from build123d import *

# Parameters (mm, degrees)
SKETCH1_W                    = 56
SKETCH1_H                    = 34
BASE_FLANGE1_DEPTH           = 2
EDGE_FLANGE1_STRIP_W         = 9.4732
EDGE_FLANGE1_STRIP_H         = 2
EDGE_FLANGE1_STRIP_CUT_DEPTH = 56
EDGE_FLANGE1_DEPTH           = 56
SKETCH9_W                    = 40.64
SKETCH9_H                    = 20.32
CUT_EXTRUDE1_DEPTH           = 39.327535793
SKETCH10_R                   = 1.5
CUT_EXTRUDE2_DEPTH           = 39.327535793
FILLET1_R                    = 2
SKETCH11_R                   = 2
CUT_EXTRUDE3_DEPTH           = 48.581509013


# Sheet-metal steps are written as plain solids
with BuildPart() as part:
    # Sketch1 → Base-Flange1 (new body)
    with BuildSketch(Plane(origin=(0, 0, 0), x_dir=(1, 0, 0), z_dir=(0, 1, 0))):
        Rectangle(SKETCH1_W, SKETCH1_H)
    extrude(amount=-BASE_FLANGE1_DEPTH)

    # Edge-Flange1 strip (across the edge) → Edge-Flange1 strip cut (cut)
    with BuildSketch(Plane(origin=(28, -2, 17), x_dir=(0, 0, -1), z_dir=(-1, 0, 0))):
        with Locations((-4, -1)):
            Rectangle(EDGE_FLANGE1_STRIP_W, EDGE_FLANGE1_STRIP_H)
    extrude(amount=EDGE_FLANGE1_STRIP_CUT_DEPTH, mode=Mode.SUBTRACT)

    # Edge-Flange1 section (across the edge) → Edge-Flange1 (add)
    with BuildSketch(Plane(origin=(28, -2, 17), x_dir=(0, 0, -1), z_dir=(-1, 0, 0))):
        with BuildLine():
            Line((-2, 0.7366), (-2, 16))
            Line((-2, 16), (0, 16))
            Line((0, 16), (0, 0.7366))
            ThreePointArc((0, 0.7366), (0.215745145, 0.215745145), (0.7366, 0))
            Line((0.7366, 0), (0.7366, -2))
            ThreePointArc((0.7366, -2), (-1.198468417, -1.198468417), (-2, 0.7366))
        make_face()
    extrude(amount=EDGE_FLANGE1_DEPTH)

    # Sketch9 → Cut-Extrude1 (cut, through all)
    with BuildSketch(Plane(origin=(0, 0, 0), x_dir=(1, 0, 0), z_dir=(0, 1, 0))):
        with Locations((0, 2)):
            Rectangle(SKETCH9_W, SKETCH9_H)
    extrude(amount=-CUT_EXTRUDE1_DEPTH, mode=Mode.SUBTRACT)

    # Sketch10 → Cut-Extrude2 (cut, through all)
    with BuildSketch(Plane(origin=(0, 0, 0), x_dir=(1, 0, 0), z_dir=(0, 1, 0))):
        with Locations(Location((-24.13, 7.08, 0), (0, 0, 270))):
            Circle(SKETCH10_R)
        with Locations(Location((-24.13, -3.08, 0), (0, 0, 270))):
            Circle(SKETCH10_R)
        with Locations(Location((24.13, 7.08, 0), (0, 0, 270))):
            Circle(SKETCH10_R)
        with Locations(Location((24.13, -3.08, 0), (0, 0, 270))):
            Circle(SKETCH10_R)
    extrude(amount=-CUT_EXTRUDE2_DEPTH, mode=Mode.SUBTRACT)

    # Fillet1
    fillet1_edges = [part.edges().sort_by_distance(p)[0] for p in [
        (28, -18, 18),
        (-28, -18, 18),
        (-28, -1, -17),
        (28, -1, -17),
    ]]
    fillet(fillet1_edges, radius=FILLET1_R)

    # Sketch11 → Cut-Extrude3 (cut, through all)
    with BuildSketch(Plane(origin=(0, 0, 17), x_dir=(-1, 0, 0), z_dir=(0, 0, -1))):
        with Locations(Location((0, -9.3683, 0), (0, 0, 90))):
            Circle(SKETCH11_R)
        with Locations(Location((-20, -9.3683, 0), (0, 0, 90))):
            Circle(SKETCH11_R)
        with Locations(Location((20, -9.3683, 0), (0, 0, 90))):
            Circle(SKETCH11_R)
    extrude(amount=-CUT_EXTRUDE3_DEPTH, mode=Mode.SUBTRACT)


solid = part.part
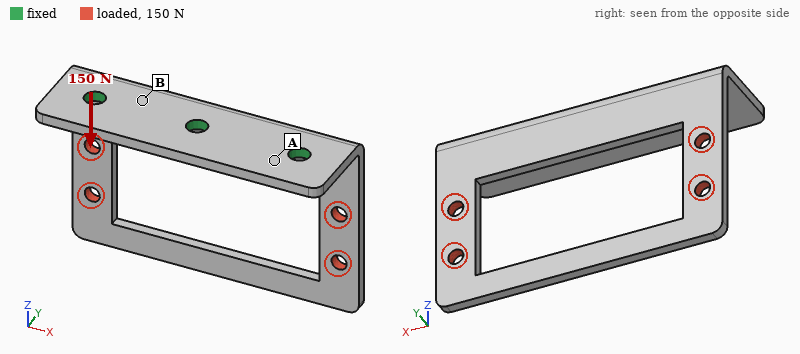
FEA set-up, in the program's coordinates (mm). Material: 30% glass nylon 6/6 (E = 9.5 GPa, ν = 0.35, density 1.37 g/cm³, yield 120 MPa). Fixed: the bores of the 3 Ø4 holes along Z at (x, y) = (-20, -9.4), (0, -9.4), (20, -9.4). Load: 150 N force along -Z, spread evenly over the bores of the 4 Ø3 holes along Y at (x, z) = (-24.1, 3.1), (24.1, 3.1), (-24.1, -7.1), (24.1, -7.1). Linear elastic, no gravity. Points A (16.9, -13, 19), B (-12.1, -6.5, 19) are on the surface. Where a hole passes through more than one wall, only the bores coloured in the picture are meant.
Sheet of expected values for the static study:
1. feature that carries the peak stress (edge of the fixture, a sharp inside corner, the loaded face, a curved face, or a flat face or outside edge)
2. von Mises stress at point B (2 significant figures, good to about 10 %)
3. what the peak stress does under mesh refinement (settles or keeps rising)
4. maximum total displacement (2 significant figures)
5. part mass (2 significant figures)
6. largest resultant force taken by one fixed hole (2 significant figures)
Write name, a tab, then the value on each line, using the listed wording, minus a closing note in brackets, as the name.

feature that carries the peak stress	edge of the fixture
von Mises stress at point B	11 MPa
what the peak stress does under mesh refinement	keeps rising
maximum total displacement	0.49 mm
part mass	5.4 g
largest resultant force taken by one fixed hole	65 N
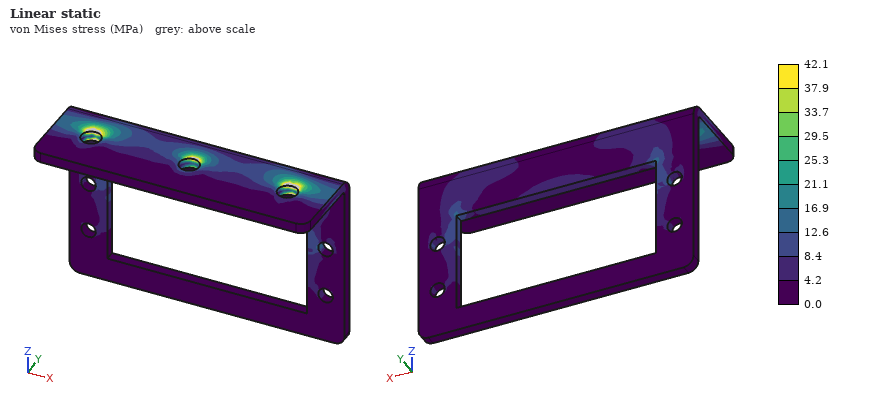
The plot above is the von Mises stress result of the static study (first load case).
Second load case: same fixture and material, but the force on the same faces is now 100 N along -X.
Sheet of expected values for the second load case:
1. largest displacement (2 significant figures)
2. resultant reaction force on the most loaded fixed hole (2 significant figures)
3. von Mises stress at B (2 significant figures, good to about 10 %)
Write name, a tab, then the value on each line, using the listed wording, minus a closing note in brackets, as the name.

largest displacement	0.36 mm
resultant reaction force on the most loaded fixed hole	60 N
von Mises stress at B	4.3 MPa
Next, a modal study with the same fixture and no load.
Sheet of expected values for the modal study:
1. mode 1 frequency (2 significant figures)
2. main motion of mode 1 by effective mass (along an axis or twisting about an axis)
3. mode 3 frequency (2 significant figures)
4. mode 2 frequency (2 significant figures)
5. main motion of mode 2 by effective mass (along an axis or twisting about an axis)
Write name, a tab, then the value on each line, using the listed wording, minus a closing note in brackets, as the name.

mode 1 frequency	470 Hz
main motion of mode 1 by effective mass	along Y
mode 3 frequency	1900 Hz
mode 2 frequency	850 Hz
main motion of mode 2 by effective mass	twisting about Z
